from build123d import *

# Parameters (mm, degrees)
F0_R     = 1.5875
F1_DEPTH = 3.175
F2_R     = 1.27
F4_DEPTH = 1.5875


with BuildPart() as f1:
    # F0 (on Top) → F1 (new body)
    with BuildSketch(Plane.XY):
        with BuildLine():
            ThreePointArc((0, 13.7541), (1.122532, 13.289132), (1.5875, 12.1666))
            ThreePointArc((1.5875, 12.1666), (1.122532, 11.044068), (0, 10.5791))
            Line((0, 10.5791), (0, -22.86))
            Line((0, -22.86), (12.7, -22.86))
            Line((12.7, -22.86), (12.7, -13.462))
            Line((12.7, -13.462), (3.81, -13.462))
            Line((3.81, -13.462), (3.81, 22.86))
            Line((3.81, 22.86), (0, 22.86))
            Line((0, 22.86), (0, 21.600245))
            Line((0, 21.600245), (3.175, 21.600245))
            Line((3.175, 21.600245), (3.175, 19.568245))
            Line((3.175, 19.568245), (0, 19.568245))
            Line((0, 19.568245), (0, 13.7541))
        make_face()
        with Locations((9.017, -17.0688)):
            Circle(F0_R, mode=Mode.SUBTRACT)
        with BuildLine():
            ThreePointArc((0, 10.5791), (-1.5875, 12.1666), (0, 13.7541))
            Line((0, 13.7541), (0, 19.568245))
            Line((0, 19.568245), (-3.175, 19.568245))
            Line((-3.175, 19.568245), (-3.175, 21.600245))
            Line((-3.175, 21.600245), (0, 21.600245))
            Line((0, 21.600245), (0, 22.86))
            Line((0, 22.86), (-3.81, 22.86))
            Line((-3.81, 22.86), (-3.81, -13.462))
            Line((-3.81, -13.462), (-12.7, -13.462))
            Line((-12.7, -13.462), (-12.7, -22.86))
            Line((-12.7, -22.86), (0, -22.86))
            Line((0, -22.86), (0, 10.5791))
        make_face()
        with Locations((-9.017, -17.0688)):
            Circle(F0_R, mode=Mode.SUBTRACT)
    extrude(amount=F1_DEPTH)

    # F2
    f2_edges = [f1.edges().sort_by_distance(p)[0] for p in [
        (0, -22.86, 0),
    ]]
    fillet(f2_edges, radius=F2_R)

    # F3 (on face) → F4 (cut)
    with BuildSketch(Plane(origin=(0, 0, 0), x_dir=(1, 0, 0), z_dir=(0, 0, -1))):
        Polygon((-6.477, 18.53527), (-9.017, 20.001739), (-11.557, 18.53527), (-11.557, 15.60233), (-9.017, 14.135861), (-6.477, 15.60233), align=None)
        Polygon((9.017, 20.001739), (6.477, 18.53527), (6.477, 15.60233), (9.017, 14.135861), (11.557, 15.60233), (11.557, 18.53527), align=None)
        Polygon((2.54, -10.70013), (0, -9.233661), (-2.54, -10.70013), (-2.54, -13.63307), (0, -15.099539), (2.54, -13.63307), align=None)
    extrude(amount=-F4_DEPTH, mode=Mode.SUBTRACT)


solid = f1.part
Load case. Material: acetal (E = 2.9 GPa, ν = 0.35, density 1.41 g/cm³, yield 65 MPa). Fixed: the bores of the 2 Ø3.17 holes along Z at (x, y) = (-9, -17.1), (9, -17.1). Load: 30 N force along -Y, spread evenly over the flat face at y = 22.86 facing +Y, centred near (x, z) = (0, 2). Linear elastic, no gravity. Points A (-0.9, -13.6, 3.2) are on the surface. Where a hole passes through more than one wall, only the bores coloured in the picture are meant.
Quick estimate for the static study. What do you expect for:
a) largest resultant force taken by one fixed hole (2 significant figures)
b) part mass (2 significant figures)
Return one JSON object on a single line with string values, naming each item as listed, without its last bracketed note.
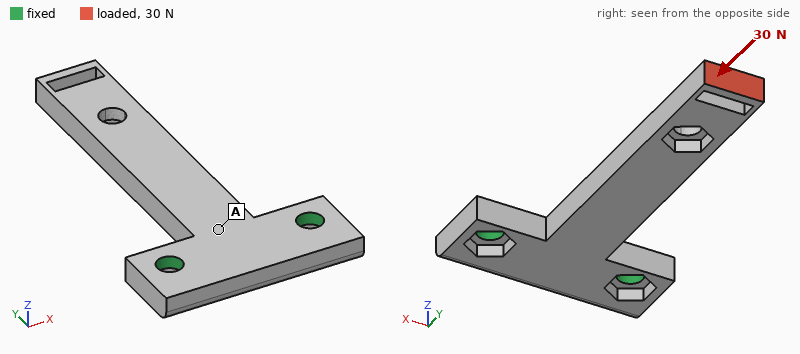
{"largest resultant force taken by one fixed hole": "15 N", "part mass": "2.0 g"}
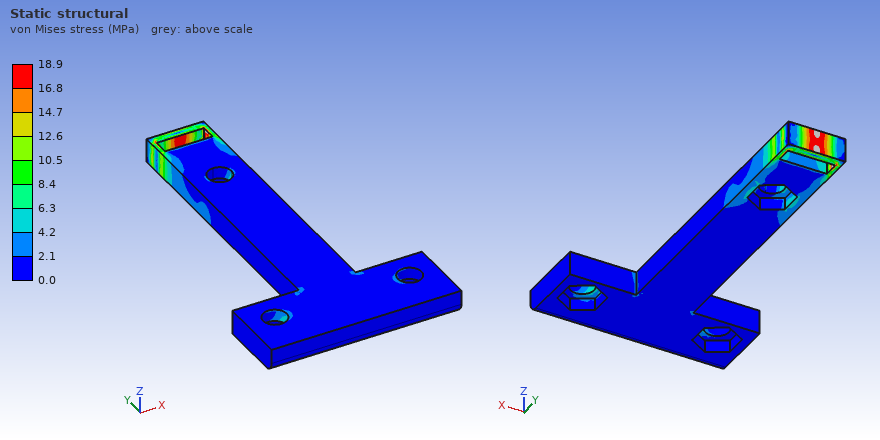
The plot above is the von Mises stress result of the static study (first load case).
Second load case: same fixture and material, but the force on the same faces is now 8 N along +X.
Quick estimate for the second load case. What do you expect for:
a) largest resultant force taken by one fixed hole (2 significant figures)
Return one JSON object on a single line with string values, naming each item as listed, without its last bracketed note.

{"largest resultant force taken by one fixed hole": "20 N"}
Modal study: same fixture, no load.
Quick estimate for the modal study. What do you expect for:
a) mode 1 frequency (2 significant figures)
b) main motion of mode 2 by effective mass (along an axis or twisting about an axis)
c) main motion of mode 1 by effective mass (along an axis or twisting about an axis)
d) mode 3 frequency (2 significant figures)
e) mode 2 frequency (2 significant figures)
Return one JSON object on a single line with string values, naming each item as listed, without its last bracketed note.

{"mode 1 frequency": "470 Hz", "main motion of mode 2 by effective mass": "along X", "main motion of mode 1 by effective mass": "along Z", "mode 3 frequency": "2500 Hz", "mode 2 frequency": "1300 Hz"}
